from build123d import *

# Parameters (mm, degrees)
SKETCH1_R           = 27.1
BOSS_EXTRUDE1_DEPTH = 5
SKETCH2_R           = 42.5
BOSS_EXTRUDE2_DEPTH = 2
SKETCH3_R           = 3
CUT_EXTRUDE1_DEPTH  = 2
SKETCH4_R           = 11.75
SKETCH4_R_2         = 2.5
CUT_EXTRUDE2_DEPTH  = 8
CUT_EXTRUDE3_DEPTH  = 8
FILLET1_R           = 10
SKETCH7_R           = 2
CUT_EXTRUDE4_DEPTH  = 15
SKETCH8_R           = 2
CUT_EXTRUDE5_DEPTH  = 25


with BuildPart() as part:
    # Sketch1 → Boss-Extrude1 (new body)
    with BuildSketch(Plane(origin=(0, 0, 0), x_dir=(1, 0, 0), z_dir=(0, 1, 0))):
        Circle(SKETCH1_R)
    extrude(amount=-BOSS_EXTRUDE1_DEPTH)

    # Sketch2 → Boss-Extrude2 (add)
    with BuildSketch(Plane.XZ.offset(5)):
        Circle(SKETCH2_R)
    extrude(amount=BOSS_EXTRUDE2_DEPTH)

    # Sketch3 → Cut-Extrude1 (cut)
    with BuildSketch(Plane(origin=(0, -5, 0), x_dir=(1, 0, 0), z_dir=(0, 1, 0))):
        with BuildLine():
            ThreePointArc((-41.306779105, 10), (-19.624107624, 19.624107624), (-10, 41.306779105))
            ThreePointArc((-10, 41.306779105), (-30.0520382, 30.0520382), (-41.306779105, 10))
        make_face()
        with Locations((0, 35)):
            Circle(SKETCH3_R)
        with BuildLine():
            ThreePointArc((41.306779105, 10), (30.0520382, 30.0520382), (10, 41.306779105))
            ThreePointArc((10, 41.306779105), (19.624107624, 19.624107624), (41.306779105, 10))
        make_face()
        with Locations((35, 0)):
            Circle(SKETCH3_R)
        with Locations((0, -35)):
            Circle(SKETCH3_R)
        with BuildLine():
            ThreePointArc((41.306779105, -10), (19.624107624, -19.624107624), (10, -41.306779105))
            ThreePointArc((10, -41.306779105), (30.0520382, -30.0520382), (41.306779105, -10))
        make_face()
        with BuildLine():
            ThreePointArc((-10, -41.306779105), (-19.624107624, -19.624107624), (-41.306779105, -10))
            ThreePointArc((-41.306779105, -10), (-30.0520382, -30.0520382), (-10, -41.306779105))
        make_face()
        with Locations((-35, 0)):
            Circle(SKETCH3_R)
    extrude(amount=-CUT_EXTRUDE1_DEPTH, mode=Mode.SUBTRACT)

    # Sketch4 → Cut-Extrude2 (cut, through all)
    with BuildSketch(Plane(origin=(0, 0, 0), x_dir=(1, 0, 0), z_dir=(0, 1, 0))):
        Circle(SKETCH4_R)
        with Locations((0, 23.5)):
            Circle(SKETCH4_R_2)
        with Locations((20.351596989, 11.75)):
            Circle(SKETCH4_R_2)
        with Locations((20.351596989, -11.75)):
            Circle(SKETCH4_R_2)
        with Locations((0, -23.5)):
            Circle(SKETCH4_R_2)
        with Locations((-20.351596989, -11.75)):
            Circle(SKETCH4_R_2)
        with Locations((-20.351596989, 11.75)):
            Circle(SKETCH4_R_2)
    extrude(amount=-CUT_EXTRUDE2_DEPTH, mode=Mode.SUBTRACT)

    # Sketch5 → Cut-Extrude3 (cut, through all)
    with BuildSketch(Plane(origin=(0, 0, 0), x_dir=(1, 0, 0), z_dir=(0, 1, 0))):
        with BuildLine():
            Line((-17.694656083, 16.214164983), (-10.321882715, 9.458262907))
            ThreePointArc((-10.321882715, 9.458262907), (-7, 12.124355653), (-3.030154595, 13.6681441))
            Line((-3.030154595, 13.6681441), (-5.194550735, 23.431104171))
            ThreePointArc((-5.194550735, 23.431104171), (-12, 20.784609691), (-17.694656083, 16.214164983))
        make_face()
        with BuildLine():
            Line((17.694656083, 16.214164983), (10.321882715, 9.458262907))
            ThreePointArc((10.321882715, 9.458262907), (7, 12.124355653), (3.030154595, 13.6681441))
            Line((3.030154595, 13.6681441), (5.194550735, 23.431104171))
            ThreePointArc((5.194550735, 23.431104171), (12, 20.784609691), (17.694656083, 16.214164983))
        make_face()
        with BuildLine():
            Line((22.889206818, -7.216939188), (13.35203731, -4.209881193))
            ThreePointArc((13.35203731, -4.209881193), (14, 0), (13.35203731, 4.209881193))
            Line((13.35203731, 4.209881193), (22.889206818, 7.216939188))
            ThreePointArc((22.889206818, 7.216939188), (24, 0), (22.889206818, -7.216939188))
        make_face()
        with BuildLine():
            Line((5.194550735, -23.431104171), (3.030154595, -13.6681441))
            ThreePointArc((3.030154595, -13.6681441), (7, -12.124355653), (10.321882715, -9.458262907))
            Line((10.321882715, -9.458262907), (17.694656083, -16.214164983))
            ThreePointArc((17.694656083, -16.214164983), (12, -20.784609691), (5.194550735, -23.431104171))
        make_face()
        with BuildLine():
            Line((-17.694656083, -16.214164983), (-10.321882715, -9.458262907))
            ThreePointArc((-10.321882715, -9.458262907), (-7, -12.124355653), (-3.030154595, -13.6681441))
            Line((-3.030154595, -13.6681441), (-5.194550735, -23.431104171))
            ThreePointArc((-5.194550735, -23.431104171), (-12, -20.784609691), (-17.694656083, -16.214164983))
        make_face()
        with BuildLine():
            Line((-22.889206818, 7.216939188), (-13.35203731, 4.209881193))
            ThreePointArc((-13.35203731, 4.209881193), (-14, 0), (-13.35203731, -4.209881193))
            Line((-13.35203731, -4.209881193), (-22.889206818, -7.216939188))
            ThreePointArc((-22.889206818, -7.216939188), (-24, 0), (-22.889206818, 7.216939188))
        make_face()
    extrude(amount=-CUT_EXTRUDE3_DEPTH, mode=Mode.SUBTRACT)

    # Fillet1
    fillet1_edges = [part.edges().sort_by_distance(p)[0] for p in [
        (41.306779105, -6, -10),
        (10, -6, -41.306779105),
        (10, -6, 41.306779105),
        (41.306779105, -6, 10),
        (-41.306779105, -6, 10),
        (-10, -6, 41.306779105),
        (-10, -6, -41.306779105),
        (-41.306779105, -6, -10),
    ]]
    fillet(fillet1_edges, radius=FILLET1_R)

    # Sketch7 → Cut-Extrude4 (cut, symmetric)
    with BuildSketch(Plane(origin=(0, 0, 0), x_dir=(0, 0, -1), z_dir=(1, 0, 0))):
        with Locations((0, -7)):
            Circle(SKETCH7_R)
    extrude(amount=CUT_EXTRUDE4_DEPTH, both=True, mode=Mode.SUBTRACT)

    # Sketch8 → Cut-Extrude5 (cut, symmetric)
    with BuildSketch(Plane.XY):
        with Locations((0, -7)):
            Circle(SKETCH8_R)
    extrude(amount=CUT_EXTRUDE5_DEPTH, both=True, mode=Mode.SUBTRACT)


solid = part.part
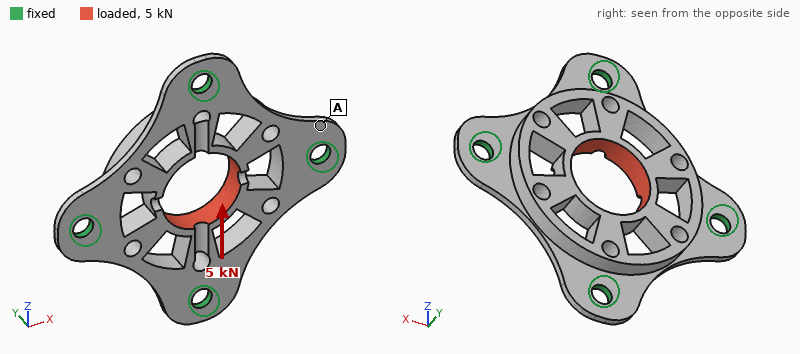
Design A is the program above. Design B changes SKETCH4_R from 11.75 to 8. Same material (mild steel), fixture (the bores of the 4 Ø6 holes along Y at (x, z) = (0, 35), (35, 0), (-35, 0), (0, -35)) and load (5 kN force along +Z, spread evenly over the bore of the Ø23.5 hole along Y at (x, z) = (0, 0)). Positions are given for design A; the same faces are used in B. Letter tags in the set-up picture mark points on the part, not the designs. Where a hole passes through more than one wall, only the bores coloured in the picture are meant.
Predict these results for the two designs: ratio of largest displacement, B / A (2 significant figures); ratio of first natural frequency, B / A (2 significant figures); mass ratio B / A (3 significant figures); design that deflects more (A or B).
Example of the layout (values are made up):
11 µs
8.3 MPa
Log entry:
0.56
0.93
1.15
A
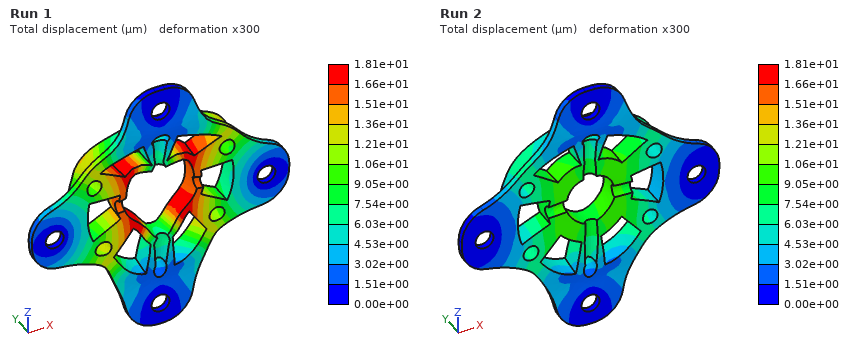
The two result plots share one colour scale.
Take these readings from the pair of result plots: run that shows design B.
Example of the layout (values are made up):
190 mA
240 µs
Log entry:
Run 2
